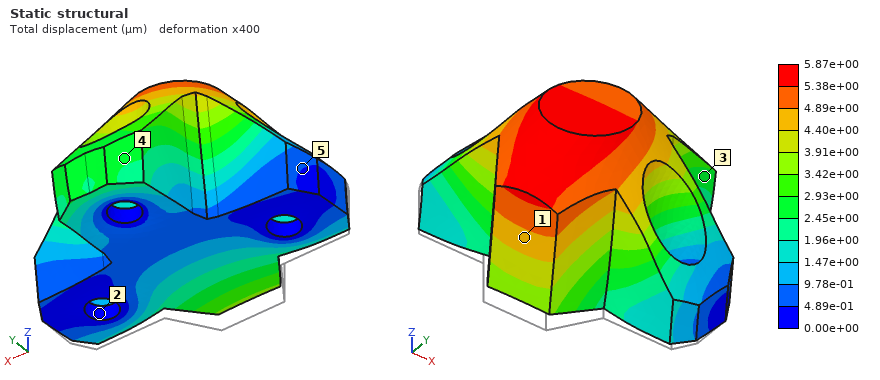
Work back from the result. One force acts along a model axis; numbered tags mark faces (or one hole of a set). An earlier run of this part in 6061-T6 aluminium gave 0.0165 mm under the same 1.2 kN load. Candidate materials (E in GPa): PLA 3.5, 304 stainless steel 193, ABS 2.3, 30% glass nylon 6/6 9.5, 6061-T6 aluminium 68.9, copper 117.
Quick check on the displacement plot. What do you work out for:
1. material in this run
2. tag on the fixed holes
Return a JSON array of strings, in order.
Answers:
["304 stainless steel", "2"]
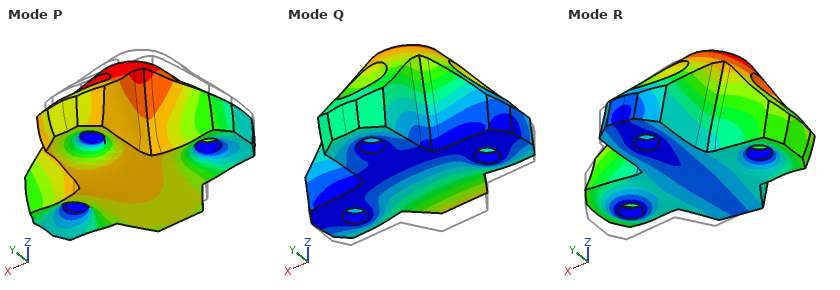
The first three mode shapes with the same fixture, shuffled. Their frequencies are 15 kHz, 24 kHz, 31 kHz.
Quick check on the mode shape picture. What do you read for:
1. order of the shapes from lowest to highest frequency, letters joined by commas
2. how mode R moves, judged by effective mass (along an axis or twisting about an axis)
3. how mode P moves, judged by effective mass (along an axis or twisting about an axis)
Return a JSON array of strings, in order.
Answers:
["Q, R, P", "along X", "along Z"]
